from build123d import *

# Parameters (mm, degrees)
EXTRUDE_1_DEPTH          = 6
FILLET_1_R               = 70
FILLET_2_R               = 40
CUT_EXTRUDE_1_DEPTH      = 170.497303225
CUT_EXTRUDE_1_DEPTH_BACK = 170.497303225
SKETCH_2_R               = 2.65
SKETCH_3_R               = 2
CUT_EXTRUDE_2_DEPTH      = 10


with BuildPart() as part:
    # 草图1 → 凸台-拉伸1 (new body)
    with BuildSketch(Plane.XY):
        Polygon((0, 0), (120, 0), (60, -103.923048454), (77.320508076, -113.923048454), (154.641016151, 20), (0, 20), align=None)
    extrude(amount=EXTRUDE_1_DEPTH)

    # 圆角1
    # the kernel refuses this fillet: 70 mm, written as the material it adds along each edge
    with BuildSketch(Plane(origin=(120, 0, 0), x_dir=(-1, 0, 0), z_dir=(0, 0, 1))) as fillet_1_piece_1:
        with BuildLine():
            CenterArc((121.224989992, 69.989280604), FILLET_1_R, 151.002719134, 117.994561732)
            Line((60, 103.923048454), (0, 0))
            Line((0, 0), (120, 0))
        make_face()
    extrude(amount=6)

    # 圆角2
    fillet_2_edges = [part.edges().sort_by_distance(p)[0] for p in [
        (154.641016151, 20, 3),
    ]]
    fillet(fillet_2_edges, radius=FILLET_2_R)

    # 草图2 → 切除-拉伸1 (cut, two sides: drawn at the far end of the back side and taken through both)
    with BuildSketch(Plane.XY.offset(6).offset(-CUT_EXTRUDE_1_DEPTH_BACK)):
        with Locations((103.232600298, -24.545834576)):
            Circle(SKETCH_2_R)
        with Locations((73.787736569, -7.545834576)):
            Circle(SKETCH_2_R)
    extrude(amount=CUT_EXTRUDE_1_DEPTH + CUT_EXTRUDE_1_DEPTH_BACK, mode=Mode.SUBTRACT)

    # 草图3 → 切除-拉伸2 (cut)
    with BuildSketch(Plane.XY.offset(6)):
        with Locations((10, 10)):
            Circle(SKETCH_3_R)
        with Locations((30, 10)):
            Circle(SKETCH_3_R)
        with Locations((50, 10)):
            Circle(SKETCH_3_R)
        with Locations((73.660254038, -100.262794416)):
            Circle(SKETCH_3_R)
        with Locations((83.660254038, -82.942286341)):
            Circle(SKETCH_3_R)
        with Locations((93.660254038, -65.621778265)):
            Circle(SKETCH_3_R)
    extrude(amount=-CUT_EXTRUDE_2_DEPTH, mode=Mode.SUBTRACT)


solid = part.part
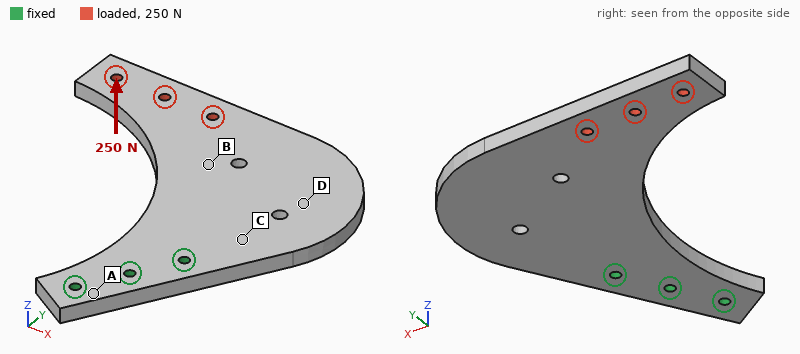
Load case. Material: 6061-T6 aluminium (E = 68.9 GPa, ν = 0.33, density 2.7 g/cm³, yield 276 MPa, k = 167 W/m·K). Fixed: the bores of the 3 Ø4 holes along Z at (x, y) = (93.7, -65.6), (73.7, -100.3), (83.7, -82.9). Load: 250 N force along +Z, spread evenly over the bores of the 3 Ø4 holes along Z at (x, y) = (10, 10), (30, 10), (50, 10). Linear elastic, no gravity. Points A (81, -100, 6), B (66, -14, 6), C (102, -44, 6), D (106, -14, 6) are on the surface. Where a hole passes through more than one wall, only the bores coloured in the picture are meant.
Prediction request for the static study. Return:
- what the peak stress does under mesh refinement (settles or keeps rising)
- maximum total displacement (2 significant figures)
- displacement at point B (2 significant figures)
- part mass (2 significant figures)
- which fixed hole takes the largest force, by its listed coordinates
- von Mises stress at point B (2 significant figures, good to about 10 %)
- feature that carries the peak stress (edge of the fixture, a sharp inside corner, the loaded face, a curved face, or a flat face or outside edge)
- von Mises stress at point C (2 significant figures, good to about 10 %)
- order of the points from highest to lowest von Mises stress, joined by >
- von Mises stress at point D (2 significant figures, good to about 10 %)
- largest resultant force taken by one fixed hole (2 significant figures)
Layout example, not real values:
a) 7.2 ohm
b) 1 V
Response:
a) keeps rising
b) 2.2 mm
c) 0.64 mm
d) 120 g
e) (93.7, -65.6)
f) 39 MPa
g) edge of the fixture
h) 54 MPa
i) C > B > D > A
j) 28 MPa
k) 470 N
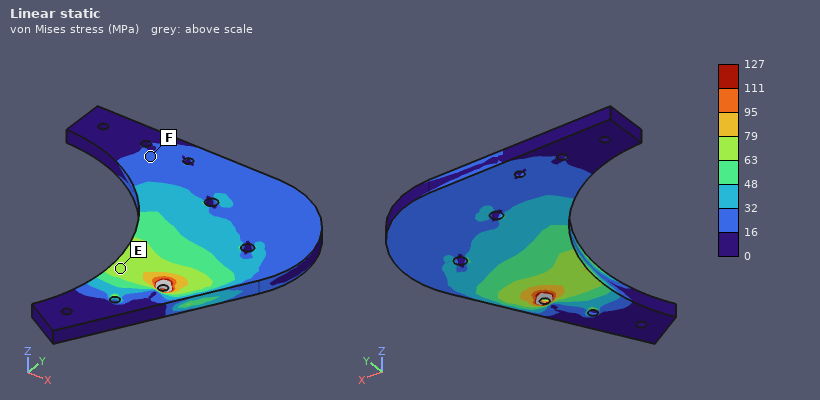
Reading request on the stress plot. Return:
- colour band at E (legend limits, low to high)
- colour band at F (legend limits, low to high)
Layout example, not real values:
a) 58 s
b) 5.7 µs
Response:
a) 63 to 79 MPa
b) 16 to 32 MPa
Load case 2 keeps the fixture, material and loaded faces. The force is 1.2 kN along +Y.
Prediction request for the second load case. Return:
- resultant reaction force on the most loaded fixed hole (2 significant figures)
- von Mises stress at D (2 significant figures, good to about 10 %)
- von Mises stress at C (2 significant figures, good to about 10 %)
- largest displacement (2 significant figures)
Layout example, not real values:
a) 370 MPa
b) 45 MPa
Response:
a) 2.2 kN
b) 8.1 MPa
c) 12 MPa
d) 0.24 mm
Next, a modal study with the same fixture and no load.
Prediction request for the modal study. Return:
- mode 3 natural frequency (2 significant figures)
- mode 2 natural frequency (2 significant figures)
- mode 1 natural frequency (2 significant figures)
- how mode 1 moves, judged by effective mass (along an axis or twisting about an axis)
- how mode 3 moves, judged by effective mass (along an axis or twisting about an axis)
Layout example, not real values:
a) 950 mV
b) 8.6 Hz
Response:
a) 1600 Hz
b) 810 Hz
c) 360 Hz
d) along Z
e) along X
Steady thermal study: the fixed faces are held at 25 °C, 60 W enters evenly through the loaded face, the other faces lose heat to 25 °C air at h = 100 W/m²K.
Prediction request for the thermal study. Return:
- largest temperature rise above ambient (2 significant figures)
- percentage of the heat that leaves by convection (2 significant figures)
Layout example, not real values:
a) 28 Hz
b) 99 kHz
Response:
a) 77 K
b) 73 %
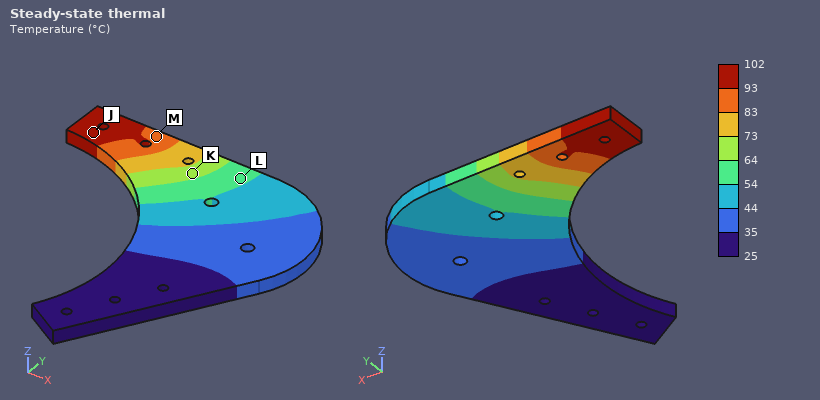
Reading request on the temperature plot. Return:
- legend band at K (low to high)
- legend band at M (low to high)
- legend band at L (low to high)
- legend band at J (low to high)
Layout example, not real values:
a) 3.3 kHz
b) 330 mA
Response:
a) 64 to 73 °C
b) 83 to 93 °C
c) 54 to 64 °C
d) 93 to 102 °C
